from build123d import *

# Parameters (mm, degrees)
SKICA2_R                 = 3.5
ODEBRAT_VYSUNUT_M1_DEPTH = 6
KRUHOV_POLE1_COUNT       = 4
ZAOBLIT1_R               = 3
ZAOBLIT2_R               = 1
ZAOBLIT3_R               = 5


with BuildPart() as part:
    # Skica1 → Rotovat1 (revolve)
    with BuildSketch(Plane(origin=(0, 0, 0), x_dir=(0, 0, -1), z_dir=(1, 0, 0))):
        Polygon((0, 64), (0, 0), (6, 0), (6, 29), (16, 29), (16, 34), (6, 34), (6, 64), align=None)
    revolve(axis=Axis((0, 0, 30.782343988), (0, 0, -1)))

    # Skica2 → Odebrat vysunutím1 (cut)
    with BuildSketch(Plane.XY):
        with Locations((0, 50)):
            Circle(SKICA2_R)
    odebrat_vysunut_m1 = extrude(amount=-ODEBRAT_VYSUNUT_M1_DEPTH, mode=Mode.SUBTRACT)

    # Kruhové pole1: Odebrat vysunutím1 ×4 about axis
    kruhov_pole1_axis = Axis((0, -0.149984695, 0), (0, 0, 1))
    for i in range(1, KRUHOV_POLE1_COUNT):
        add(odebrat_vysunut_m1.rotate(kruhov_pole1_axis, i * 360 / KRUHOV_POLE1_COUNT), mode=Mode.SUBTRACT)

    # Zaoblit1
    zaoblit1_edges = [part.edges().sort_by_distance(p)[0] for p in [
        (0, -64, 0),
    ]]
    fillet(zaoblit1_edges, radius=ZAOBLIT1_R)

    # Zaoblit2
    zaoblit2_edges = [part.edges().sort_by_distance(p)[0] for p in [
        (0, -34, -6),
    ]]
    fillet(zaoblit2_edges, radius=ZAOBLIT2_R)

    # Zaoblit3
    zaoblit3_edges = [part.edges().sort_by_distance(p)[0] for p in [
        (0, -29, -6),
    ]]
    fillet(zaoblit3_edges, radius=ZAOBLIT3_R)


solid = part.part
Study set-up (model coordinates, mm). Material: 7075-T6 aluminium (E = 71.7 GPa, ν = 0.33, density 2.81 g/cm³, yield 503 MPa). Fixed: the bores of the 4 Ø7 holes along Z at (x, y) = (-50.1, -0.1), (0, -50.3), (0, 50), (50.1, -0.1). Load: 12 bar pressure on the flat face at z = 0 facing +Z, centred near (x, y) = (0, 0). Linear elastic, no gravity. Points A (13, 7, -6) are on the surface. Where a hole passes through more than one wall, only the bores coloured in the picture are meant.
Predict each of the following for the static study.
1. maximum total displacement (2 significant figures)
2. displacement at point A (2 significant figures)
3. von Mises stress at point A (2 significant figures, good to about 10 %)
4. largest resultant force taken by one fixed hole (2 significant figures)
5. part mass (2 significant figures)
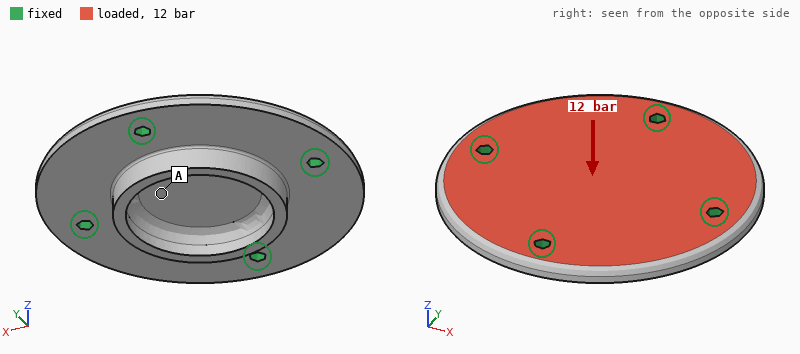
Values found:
87 µm
67 µm
16 MPa
3.5 kN
240 g
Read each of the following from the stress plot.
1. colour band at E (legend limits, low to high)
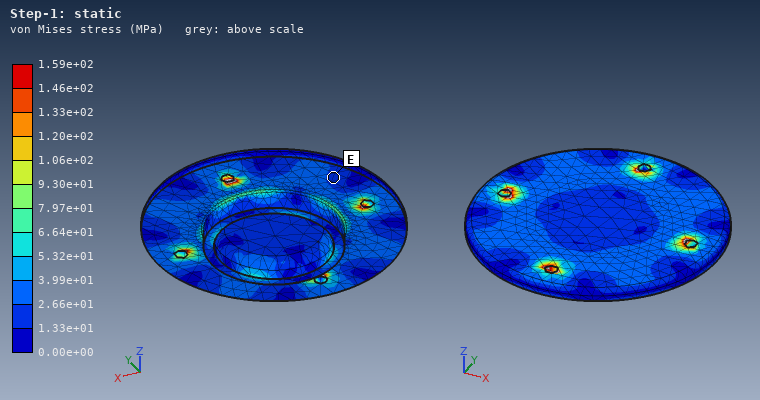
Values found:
1.33e+01 to 2.66e+01 MPa
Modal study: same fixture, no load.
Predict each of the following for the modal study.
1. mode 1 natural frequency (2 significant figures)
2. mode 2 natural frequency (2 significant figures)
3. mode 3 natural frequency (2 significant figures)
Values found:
4700 Hz
5000 Hz
5000 Hz
